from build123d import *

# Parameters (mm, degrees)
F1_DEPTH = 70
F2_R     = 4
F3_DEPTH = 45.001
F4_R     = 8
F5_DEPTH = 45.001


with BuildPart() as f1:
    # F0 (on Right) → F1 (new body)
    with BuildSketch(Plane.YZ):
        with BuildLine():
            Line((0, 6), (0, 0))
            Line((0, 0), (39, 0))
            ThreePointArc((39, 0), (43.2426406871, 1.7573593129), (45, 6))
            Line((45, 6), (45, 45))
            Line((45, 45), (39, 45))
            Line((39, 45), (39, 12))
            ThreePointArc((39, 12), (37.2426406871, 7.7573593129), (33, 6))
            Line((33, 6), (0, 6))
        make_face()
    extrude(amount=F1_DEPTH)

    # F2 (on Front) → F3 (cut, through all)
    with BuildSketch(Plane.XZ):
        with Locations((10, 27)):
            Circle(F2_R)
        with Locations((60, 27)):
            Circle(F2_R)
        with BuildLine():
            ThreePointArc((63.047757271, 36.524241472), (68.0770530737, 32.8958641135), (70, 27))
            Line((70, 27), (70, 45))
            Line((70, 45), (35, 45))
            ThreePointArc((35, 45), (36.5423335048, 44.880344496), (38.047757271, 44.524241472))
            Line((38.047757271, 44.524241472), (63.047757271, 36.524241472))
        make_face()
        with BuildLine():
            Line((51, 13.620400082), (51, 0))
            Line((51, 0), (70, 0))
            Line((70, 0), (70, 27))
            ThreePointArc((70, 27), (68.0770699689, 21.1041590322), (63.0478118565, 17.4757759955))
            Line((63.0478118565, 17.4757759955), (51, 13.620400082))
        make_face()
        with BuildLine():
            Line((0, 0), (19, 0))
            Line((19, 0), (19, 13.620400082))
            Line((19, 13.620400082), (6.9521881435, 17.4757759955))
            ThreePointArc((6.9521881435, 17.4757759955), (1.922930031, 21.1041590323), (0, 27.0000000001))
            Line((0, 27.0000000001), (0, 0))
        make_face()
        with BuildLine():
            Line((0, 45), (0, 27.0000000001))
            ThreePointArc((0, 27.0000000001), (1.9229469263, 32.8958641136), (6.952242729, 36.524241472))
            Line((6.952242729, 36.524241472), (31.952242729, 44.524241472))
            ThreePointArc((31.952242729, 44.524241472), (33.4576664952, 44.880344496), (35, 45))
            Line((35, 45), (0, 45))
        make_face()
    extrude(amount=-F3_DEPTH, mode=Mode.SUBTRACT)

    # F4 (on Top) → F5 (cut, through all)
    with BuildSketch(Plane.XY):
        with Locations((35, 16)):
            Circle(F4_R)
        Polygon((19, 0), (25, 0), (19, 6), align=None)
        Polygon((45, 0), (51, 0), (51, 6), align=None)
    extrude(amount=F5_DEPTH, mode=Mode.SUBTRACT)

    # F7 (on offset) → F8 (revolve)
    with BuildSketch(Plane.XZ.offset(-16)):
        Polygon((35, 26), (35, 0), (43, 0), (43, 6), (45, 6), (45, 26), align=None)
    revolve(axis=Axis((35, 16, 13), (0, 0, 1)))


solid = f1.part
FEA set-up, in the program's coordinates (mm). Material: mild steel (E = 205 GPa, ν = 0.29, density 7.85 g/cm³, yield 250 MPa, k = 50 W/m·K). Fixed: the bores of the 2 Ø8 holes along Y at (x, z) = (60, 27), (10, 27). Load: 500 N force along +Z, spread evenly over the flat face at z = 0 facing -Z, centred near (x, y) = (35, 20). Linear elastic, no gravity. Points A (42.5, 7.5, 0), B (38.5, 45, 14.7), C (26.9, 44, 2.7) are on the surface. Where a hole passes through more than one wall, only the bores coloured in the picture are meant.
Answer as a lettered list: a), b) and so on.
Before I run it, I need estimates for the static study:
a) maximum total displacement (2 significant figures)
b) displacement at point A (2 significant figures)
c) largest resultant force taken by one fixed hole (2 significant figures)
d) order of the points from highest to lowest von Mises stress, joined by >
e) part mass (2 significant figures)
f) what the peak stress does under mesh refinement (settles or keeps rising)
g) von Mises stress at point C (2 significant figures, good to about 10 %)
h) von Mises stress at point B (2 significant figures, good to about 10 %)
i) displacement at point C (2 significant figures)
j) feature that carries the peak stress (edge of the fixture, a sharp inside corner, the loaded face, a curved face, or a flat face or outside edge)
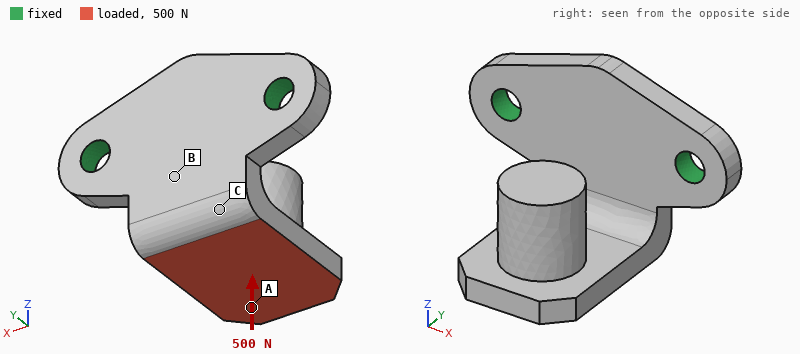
a) 0.10 mm
b) 0.086 mm
c) 260 N
d) B > C > A
e) 200 g
f) keeps rising
g) 14 MPa
h) 43 MPa
i) 0.026 mm
j) a sharp inside corner
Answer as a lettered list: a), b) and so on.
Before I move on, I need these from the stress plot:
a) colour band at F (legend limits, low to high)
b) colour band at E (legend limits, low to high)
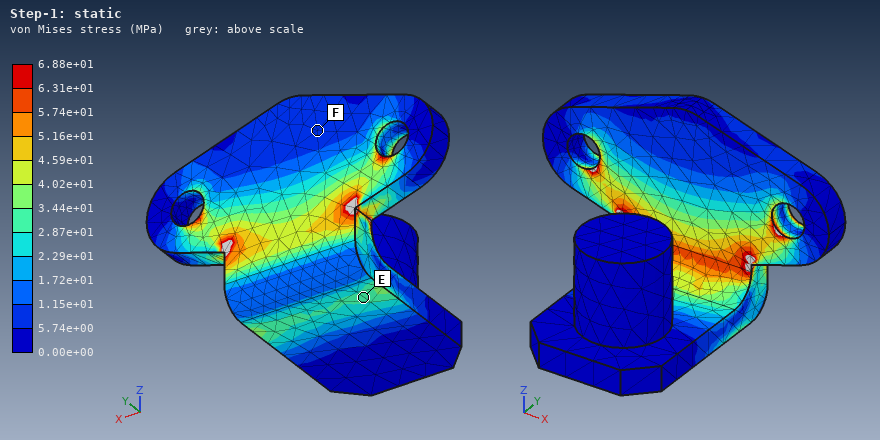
a) 5.74e+00 to 1.15e+01 MPa
b) 2.87e+01 to 3.44e+01 MPa
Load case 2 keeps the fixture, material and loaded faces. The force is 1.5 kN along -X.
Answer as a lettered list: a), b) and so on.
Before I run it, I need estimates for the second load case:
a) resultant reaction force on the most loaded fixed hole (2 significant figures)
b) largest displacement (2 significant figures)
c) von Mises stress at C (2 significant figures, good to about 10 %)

a) 1.4 kN
b) 73 µm
c) 37 MPa
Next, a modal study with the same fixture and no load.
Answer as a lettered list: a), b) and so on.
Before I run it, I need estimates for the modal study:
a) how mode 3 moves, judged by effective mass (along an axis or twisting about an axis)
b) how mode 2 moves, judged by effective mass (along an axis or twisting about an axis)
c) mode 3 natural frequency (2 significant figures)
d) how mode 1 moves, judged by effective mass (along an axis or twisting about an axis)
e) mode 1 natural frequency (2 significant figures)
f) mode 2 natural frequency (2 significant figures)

a) along Y
b) along X
c) 3100 Hz
d) along Z
e) 1200 Hz
f) 2200 Hz
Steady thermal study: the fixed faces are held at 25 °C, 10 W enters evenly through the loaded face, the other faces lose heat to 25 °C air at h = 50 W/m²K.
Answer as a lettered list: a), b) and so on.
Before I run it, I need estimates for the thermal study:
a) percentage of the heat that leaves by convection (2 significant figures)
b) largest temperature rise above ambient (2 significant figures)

a) 45 %
b) 26 K
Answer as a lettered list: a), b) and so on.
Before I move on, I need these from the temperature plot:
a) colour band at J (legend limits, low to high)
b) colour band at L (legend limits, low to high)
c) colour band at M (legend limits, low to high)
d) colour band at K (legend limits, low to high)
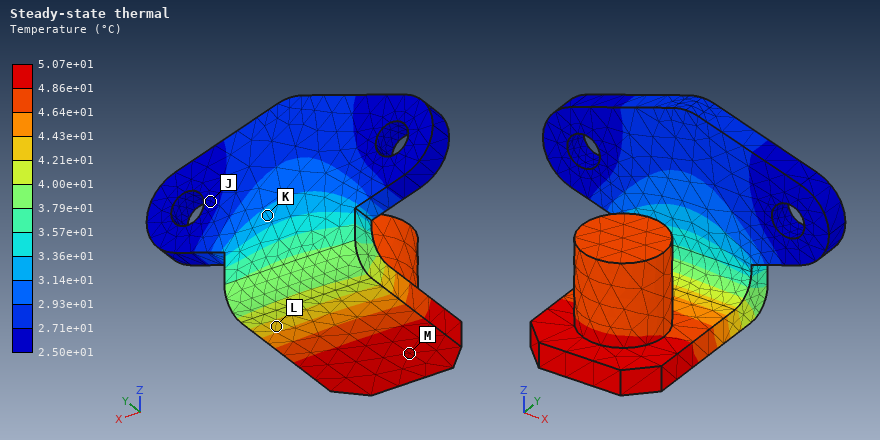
a) 2.50e+01 to 2.71e+01 °C
b) 4.21e+01 to 4.43e+01 °C
c) 4.86e+01 to 5.07e+01 °C
d) 3.14e+01 to 3.36e+01 °C
